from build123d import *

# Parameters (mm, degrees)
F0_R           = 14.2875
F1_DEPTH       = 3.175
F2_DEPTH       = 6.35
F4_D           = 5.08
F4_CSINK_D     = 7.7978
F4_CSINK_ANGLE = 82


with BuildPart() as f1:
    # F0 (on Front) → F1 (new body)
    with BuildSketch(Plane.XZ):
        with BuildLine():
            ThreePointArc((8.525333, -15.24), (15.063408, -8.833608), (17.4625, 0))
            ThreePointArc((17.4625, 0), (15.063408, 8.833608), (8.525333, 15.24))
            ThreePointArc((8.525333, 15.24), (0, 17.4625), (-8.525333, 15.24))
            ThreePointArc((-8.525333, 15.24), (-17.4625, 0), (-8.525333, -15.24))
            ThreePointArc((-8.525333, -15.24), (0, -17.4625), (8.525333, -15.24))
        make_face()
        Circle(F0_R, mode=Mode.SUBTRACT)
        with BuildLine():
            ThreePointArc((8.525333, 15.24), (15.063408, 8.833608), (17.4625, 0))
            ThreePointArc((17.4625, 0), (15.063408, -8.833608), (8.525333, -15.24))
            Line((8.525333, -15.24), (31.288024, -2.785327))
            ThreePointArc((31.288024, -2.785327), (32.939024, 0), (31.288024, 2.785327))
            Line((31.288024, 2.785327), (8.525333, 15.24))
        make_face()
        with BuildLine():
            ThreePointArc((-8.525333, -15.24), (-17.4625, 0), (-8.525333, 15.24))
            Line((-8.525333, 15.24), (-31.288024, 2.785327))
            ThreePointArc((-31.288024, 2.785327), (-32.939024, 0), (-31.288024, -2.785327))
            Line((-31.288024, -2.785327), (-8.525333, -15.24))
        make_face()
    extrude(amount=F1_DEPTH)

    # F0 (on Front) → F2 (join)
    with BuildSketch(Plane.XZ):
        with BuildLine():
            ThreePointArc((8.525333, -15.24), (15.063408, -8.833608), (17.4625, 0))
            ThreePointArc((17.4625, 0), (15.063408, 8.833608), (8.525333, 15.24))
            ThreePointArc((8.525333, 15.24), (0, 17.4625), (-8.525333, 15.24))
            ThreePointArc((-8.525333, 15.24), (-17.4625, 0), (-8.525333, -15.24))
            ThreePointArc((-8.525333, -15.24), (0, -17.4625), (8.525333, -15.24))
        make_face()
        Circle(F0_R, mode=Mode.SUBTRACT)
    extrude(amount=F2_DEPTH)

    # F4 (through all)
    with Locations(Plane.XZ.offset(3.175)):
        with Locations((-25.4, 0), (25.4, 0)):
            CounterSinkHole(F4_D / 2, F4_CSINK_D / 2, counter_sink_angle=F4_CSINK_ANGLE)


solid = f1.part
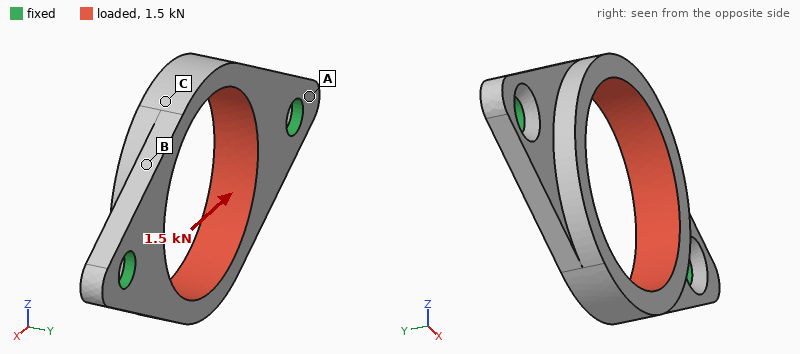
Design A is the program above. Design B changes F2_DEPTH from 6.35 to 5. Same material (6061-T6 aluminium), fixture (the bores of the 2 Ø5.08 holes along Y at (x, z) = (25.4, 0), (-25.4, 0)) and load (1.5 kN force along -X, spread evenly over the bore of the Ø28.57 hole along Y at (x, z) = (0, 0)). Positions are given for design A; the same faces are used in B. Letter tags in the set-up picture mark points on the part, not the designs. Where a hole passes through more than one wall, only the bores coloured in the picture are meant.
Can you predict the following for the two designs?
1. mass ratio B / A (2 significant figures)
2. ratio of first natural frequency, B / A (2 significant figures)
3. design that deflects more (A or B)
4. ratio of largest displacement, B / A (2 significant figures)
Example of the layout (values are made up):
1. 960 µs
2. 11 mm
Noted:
1. 0.87
2. 1.1
3. B
4. 1.1
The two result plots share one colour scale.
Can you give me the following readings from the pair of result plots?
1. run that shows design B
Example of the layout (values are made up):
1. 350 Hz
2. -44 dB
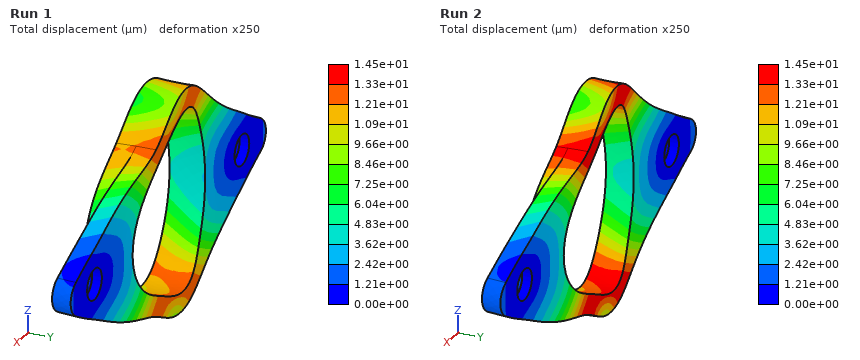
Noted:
1. Run 2
